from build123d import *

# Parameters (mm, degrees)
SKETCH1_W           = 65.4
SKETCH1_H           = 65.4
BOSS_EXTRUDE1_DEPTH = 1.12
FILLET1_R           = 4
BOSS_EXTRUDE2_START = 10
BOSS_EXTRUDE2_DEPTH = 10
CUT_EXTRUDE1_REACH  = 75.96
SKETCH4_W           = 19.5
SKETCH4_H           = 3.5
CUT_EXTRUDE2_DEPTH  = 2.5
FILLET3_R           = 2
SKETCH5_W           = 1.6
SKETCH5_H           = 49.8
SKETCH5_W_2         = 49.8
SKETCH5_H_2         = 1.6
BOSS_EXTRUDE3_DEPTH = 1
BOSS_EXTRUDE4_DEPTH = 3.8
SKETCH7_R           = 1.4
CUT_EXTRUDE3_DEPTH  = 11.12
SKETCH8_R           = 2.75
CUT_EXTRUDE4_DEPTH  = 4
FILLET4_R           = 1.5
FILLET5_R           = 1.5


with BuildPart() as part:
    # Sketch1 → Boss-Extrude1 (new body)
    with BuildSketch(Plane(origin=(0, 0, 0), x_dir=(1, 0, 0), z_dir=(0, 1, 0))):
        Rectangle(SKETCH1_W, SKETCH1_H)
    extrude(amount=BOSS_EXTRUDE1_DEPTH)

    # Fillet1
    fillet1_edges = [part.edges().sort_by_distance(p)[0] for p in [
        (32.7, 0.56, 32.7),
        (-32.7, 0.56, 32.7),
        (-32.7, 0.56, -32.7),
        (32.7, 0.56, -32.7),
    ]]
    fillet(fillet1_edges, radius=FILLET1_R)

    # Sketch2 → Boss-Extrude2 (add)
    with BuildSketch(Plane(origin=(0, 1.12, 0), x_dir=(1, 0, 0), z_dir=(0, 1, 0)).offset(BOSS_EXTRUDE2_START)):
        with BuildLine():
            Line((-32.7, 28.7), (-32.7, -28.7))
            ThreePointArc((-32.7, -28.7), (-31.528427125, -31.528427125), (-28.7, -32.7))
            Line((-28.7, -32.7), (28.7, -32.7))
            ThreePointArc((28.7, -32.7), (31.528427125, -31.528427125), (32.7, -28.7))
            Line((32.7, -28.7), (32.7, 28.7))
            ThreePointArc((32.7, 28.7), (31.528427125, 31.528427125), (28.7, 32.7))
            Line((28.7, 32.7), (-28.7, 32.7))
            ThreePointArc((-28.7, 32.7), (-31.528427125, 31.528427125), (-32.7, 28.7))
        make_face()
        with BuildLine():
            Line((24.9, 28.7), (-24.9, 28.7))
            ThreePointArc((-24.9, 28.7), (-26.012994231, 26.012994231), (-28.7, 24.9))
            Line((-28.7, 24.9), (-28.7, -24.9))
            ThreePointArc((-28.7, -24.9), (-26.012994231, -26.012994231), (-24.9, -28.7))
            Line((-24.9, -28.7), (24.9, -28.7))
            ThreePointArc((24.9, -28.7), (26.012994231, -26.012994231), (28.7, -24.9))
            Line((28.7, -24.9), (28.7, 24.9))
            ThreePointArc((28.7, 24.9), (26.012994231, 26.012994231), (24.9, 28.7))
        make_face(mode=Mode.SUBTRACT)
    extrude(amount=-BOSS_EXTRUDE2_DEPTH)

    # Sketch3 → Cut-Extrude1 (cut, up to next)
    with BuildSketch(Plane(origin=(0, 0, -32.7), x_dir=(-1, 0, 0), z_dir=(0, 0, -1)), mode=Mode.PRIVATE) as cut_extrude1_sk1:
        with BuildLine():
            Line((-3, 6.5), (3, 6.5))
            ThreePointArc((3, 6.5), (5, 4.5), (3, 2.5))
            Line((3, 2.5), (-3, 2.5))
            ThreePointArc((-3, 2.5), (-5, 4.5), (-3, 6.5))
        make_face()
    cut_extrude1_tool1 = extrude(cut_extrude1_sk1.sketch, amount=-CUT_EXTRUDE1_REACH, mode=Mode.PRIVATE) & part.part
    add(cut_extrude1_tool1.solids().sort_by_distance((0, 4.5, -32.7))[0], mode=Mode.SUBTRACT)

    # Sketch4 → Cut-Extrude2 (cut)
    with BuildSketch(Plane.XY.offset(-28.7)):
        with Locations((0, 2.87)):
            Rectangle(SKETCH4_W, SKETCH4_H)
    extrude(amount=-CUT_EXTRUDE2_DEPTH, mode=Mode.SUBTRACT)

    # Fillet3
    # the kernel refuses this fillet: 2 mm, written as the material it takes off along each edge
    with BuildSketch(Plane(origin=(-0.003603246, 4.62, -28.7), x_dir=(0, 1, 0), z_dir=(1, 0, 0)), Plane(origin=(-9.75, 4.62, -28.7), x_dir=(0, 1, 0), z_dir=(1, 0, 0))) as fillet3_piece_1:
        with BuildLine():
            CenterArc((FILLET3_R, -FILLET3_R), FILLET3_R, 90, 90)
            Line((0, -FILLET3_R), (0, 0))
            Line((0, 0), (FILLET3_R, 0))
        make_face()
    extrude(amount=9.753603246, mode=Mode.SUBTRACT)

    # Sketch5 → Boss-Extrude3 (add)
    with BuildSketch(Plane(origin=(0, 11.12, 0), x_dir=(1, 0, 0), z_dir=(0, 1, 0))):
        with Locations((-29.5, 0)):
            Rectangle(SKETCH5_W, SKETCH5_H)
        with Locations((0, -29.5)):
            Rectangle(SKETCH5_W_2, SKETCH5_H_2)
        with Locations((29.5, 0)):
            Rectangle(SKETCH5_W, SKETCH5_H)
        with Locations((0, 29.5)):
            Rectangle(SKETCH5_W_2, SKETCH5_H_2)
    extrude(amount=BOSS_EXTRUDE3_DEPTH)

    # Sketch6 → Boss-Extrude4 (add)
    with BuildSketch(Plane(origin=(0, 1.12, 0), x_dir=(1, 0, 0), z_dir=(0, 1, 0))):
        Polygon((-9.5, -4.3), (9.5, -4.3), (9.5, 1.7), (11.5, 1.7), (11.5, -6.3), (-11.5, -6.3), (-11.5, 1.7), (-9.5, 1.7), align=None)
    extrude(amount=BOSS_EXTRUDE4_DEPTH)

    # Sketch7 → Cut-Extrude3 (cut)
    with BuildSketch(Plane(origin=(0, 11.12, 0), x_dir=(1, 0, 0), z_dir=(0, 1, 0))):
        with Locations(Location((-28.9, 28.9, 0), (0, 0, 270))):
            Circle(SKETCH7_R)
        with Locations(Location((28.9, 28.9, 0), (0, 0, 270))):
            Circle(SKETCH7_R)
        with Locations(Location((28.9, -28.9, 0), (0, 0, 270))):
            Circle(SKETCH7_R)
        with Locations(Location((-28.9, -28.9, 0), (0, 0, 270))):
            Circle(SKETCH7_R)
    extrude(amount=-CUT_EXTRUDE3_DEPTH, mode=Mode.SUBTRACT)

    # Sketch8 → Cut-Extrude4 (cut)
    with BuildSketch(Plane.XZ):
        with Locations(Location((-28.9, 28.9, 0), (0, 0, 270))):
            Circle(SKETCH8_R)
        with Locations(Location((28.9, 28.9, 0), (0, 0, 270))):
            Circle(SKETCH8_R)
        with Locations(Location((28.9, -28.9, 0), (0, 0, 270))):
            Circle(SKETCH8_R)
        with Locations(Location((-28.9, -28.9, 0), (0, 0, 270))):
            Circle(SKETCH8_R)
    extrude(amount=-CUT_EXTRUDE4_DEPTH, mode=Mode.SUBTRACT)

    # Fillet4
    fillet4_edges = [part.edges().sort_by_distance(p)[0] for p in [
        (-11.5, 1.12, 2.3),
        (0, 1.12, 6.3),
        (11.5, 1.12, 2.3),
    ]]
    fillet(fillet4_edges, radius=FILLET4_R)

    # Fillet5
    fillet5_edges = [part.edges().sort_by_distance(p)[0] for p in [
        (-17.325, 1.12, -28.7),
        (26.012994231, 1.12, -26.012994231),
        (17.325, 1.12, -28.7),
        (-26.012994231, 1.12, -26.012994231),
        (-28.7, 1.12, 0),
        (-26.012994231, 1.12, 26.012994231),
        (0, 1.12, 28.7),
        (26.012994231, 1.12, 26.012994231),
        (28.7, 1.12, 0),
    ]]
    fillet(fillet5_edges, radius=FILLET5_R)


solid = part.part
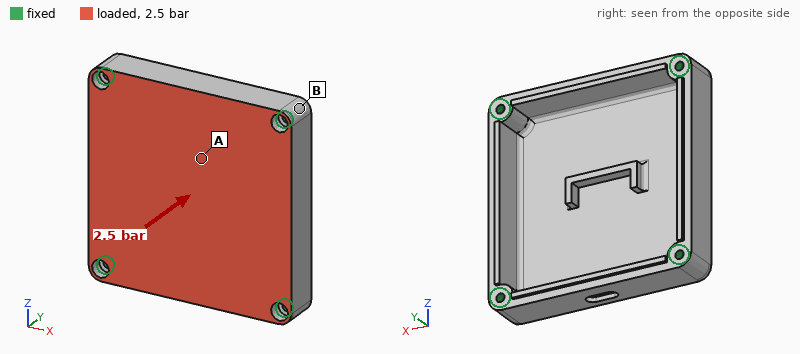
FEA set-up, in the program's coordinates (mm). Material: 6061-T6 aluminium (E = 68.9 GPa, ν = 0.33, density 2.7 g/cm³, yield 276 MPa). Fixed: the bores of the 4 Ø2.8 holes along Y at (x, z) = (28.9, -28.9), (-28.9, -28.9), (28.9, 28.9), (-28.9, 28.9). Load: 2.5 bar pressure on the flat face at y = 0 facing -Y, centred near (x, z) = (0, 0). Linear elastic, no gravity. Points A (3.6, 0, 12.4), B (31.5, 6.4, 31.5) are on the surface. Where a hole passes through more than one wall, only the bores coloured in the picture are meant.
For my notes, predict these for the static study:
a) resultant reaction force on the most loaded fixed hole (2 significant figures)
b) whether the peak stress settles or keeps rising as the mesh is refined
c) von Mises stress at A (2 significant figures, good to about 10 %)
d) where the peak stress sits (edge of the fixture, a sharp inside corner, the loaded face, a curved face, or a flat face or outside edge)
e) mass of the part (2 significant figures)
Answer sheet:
330 N
keeps rising
47 MPa
a sharp inside corner
40 g
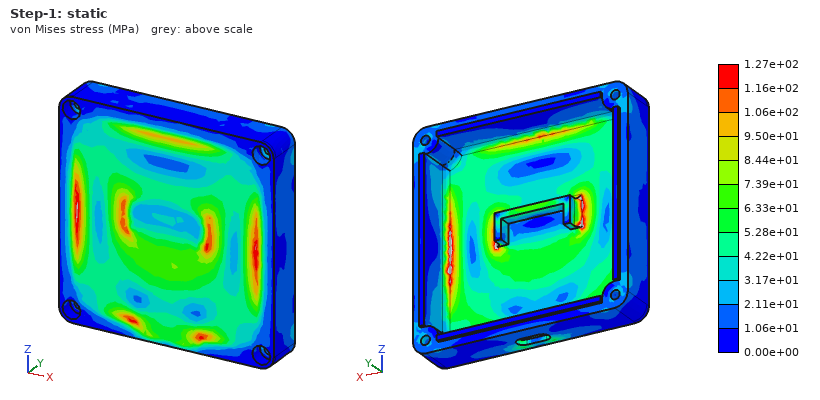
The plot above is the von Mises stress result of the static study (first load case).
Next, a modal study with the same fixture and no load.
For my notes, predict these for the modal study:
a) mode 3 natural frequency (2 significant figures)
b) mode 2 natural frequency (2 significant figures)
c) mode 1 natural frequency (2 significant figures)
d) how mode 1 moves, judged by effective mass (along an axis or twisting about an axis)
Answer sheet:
5700 Hz
5500 Hz
3000 Hz
along Y
